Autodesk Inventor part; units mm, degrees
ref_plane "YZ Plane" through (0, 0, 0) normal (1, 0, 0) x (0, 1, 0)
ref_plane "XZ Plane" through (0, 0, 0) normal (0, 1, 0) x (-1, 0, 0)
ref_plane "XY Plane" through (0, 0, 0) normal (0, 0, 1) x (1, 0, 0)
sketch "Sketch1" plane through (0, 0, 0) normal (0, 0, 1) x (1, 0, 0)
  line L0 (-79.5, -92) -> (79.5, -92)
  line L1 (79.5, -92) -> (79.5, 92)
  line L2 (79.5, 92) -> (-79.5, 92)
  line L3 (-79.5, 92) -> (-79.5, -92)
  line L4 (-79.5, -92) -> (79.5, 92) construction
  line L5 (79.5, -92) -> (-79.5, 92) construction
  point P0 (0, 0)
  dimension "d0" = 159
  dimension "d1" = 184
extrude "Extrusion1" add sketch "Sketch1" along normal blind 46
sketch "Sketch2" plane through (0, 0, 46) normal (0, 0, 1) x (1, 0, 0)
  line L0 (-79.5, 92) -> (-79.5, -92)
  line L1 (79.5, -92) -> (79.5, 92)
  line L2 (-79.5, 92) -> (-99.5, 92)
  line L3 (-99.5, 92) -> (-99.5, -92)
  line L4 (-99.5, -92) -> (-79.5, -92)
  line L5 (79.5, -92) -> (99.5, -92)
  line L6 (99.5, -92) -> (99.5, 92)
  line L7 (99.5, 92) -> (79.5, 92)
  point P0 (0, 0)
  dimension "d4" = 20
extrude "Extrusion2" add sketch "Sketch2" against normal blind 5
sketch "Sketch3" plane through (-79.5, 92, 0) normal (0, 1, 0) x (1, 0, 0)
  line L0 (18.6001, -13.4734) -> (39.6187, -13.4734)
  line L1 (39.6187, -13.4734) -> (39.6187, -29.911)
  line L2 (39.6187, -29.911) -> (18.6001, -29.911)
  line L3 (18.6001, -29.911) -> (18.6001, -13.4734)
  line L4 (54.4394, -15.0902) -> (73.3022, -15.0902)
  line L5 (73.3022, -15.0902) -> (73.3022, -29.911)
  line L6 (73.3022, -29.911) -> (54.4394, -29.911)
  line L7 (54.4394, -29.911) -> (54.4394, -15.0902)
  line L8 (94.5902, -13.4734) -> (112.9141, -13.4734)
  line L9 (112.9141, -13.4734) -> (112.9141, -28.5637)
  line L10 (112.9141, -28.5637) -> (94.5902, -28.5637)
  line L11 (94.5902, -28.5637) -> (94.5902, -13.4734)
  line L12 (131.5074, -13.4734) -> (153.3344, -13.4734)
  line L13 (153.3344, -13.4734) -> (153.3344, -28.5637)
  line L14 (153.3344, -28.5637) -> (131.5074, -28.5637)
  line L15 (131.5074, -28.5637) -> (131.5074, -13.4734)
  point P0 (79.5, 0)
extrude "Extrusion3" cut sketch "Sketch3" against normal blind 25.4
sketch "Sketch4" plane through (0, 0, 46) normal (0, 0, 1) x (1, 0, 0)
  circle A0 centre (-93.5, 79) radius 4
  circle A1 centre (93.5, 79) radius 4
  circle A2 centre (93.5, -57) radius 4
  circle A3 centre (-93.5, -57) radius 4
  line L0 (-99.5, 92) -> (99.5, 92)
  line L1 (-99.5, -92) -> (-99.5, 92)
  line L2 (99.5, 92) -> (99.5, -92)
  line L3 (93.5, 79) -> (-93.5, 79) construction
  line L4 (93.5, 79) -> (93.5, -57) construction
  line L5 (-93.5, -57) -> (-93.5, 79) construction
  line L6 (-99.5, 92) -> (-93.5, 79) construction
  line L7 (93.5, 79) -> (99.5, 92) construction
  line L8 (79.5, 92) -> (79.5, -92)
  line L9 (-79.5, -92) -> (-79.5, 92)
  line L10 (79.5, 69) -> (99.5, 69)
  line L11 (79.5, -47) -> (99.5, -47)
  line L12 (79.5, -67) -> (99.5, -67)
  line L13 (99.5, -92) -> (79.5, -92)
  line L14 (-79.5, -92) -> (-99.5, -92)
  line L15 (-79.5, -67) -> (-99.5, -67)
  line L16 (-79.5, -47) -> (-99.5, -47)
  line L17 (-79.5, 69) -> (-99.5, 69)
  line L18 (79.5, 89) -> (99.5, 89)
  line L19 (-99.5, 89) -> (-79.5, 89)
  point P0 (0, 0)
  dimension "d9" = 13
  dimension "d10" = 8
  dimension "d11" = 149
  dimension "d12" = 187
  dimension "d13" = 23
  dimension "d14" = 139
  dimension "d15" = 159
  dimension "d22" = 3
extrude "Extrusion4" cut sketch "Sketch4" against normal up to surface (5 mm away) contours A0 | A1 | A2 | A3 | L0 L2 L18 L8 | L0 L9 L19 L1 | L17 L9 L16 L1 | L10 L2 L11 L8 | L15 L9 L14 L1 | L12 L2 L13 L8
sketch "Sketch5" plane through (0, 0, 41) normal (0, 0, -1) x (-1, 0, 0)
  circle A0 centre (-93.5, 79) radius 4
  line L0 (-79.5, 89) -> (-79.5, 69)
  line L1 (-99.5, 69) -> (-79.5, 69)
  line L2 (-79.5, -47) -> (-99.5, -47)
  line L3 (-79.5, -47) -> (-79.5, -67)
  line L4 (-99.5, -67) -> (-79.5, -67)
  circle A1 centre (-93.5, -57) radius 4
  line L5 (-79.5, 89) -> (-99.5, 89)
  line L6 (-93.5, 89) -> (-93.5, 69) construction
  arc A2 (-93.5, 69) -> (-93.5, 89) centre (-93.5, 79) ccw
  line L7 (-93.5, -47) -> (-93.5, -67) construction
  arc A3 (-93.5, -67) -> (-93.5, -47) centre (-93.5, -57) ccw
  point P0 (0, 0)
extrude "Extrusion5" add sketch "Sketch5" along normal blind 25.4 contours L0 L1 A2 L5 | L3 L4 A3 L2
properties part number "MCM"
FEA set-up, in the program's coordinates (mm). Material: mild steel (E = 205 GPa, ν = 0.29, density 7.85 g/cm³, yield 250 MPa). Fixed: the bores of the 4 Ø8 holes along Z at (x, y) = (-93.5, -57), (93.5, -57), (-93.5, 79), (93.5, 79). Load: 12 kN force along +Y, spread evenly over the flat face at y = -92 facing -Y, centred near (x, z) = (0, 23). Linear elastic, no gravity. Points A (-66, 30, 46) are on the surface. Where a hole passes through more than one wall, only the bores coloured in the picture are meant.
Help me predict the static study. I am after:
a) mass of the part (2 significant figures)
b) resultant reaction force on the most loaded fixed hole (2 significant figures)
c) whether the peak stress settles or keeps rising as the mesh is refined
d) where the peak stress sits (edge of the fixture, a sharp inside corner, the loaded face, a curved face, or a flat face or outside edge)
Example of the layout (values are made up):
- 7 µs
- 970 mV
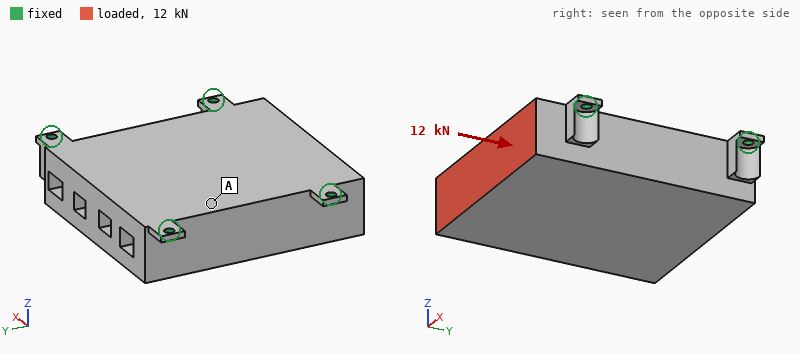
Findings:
- 10 kg
- 3.9 kN
- keeps rising
- edge of the fixture
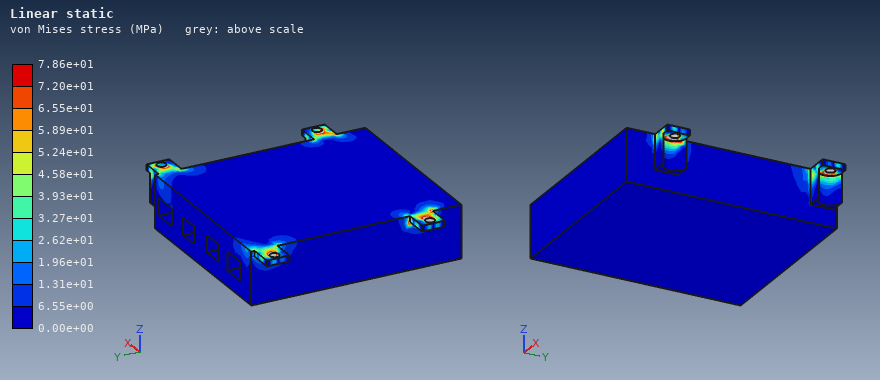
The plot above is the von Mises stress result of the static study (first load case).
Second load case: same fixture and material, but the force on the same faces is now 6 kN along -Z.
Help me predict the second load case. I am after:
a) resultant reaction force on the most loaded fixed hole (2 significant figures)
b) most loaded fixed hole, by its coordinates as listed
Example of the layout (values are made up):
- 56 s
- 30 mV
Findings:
- 5.2 kN
- (93.5, -57)
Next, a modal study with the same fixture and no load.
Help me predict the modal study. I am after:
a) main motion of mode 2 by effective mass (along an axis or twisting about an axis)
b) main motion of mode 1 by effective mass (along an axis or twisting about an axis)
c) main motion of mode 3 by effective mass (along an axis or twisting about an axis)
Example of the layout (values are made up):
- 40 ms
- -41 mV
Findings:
- along Y
- along Z
- along Y
